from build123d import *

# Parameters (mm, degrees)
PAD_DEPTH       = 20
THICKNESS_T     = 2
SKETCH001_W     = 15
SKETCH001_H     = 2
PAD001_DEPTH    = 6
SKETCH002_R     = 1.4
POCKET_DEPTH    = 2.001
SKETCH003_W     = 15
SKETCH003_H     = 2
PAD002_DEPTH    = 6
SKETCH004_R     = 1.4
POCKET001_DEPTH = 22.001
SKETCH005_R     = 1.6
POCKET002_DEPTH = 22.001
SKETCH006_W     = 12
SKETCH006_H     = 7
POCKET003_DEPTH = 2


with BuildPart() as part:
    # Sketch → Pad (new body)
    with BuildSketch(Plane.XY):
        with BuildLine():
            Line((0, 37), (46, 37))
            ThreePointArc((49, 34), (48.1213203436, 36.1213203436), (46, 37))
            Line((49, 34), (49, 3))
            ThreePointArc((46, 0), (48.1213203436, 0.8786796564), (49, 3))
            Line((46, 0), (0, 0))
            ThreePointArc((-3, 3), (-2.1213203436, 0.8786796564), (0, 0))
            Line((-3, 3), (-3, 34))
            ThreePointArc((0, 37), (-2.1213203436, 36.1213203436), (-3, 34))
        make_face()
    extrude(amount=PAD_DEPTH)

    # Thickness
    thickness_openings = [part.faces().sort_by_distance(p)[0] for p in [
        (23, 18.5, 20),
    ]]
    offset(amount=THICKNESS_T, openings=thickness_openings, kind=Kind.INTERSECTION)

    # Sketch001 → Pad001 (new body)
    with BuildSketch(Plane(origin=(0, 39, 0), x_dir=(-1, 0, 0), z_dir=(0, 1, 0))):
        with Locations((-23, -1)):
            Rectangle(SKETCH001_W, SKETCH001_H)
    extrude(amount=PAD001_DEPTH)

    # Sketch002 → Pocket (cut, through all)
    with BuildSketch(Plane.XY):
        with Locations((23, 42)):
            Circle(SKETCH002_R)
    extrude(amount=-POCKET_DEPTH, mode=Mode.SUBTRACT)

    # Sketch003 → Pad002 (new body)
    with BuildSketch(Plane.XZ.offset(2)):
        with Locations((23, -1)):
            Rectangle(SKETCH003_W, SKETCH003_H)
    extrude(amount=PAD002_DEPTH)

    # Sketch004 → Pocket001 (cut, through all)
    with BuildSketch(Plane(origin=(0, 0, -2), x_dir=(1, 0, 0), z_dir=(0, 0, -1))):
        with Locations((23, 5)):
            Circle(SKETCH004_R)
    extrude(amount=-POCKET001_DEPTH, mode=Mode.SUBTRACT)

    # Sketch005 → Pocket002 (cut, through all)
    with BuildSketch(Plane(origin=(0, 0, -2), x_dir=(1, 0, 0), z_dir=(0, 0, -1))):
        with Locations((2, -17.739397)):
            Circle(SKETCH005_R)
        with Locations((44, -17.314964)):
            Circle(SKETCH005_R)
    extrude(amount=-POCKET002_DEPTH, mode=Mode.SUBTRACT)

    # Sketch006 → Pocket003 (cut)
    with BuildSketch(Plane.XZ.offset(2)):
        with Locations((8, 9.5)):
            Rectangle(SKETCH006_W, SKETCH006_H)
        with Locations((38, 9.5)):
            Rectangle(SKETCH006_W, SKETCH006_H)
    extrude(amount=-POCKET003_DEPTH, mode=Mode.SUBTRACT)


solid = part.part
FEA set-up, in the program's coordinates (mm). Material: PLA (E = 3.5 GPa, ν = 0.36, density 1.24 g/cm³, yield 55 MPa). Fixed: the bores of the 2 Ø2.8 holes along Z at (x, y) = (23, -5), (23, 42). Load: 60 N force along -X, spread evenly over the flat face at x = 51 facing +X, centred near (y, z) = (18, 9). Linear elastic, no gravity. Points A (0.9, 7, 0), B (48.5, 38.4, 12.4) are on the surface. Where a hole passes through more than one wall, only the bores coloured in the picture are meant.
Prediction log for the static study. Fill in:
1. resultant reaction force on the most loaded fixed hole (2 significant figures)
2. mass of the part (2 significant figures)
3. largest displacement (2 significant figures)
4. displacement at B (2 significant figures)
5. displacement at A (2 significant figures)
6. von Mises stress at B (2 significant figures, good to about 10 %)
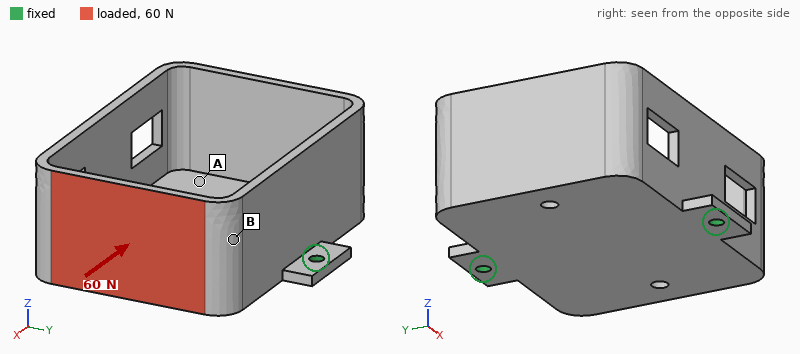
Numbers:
30 N
14 g
0.85 mm
0.50 mm
0.37 mm
4.9 MPa
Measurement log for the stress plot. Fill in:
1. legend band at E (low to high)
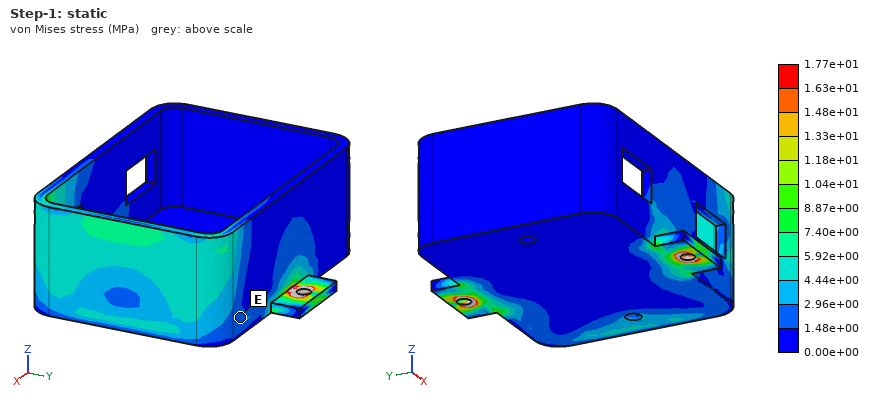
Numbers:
1.48e+00 to 2.96e+00 MPa
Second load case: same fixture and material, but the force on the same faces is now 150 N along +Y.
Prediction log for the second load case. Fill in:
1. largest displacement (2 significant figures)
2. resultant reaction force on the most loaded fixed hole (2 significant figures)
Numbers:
0.79 mm
120 N
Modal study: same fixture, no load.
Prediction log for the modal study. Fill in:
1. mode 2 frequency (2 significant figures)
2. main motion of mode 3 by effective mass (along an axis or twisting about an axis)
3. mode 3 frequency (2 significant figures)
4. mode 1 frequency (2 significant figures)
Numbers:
810 Hz
along Z
1400 Hz
370 Hz
